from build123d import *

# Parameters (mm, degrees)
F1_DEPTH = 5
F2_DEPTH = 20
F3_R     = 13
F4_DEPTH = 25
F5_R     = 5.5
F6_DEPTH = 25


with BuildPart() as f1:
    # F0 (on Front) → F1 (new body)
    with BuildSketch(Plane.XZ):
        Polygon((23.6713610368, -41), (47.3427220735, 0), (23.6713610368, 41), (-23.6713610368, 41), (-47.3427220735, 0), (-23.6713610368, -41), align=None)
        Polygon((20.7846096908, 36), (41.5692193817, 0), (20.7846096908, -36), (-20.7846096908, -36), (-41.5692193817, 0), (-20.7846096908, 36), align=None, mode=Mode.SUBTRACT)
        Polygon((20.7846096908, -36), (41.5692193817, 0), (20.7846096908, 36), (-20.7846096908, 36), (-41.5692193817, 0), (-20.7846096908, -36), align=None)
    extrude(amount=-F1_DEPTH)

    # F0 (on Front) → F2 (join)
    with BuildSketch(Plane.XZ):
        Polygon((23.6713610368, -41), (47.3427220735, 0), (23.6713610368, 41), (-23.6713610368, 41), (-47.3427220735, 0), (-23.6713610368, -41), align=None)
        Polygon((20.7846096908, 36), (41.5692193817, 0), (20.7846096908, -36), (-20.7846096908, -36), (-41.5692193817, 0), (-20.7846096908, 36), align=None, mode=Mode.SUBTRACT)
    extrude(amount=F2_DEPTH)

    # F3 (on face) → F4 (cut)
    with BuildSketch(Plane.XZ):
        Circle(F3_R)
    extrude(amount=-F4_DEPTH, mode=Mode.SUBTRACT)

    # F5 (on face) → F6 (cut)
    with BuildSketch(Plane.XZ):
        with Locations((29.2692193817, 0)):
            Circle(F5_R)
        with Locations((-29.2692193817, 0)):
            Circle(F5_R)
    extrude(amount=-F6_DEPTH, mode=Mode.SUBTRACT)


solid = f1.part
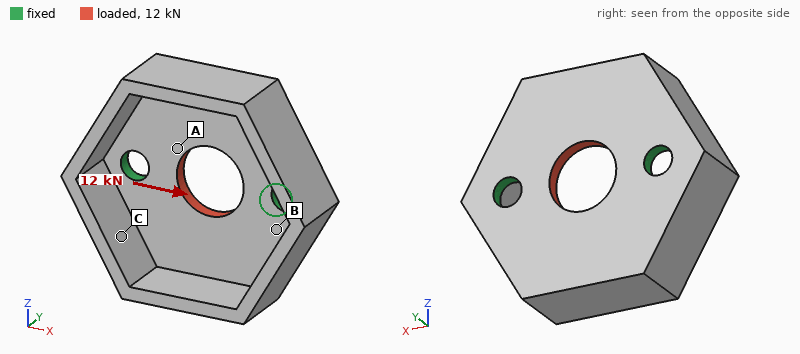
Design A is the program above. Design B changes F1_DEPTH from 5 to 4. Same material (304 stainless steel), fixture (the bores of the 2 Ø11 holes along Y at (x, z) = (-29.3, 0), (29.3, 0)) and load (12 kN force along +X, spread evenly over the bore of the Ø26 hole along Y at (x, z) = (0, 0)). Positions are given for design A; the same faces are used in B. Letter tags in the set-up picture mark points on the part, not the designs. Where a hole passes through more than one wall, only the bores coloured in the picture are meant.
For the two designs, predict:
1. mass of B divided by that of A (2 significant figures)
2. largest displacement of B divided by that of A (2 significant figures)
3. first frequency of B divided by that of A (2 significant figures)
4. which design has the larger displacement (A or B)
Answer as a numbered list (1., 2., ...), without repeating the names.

1. 0.90
2. 1.2
3. 0.82
4. B
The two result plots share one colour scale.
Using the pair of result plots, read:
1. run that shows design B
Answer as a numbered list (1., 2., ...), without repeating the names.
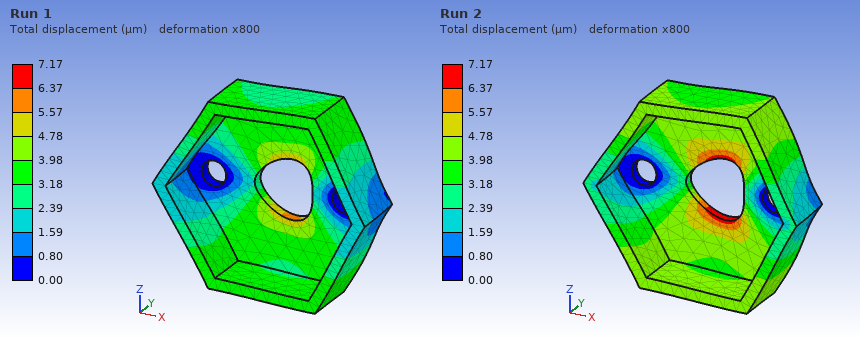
1. Run 2
